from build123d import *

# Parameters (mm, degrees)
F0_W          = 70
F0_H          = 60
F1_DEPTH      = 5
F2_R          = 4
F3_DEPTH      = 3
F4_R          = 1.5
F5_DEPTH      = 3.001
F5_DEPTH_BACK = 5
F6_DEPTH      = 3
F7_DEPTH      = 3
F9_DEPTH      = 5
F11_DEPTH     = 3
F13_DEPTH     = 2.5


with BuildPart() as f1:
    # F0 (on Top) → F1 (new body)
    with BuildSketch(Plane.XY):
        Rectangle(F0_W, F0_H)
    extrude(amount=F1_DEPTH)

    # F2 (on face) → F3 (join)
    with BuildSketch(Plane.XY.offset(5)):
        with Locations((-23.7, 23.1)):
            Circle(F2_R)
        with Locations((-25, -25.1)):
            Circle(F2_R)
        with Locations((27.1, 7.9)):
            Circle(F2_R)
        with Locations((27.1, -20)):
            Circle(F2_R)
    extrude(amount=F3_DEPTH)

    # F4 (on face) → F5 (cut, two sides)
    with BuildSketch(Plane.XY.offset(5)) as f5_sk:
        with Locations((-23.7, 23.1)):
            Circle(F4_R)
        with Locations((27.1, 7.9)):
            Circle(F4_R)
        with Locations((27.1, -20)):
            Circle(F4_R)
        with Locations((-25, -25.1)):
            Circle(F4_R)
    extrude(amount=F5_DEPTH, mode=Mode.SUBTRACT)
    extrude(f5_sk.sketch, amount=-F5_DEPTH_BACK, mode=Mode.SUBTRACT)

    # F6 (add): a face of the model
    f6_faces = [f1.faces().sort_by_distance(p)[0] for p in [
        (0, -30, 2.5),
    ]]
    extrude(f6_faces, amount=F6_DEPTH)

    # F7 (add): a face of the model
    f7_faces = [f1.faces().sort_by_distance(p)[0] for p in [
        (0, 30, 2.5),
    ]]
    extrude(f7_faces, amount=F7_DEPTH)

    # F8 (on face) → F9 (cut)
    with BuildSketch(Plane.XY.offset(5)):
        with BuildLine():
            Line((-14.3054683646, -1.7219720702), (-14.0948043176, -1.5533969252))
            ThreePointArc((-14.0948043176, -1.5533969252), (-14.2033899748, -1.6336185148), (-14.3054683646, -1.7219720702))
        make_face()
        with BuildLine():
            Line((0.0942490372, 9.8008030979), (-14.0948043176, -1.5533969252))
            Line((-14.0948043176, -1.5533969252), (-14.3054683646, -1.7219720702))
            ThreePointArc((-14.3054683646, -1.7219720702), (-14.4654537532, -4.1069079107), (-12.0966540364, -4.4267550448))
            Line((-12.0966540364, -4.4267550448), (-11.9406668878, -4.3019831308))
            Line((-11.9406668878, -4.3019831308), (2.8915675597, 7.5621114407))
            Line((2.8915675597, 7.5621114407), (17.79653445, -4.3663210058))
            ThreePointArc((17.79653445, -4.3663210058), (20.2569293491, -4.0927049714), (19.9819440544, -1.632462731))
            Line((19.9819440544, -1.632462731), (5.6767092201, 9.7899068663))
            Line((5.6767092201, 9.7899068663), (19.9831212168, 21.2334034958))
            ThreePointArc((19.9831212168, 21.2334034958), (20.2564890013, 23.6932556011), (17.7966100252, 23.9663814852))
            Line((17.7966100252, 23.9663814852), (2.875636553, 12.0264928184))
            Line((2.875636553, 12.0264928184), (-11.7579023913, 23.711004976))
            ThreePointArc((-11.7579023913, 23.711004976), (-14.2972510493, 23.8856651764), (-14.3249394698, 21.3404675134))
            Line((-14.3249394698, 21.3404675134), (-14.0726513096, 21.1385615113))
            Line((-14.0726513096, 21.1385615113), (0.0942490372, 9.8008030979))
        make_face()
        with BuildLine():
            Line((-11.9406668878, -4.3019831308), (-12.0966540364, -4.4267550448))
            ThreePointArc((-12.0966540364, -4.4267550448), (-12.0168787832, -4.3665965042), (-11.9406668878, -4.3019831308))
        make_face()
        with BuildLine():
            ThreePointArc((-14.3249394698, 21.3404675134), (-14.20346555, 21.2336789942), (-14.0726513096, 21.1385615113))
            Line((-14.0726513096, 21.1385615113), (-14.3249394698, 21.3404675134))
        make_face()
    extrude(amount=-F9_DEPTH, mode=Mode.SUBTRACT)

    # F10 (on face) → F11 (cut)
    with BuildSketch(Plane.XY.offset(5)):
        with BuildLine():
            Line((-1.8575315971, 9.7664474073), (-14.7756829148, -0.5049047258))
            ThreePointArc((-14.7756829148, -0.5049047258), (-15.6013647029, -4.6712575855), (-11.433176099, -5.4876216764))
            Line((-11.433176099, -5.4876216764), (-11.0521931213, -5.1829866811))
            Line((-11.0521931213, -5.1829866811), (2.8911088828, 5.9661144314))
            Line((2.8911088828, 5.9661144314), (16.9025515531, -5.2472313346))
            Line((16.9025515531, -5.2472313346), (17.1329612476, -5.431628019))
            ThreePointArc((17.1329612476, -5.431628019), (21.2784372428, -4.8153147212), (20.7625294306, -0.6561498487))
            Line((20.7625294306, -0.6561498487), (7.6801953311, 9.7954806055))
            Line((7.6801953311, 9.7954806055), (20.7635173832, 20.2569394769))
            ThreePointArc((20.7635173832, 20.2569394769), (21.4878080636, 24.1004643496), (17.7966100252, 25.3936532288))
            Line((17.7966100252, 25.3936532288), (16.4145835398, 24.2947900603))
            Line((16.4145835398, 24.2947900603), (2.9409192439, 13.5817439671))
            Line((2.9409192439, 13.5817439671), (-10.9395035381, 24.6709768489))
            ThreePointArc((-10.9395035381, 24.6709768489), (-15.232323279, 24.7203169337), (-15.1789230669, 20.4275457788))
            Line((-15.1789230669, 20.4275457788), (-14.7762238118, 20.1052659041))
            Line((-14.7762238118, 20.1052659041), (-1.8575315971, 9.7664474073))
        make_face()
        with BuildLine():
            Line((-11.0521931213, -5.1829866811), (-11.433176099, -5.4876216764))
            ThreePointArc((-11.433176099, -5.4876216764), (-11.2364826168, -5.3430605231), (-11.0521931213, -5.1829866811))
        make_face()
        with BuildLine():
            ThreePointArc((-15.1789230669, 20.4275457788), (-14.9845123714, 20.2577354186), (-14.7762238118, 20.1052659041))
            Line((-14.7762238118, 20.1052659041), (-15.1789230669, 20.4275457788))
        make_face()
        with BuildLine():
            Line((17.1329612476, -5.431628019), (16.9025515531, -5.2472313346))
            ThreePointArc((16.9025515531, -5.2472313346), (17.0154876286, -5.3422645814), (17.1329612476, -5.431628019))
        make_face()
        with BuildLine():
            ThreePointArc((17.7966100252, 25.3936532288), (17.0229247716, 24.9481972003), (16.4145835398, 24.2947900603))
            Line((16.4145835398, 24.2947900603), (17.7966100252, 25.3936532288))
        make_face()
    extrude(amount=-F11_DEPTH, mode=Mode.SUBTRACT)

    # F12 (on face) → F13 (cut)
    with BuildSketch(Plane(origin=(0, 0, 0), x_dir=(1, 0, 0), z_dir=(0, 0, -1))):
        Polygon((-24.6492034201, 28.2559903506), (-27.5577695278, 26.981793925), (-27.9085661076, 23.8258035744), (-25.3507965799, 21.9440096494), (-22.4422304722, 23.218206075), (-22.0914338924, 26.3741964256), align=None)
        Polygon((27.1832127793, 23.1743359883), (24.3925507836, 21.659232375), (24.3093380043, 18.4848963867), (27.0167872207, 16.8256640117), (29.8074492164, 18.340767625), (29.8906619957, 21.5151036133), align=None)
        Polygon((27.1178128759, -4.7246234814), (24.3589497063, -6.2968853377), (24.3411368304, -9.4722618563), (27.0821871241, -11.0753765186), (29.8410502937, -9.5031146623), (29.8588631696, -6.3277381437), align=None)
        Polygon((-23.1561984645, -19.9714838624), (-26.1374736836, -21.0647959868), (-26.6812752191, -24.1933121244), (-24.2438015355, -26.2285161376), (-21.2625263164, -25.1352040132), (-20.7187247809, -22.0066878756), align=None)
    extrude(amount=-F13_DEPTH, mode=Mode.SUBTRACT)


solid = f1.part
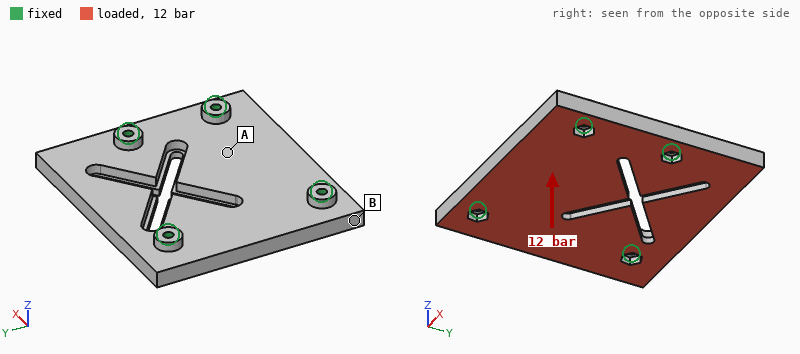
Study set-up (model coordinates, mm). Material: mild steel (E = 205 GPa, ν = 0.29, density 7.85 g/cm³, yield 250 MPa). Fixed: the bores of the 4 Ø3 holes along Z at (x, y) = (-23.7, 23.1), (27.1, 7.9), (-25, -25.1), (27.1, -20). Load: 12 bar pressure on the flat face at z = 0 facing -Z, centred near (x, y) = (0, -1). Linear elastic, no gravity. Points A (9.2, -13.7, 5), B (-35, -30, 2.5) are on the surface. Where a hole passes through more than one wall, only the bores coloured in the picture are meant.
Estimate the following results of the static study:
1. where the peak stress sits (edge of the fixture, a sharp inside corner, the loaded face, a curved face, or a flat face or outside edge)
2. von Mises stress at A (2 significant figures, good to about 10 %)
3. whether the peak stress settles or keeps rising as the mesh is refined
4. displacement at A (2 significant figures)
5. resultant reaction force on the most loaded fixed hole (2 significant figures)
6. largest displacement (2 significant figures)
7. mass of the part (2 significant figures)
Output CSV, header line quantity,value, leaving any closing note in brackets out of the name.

quantity,value
where the peak stress sits,edge of the fixture
von Mises stress at A,31 MPa
whether the peak stress settles or keeps rising as the mesh is refined,keeps rising
displacement at A,19 µm
resultant reaction force on the most loaded fixed hole,1.6 kN
largest displacement,45 µm
mass of the part,170 g
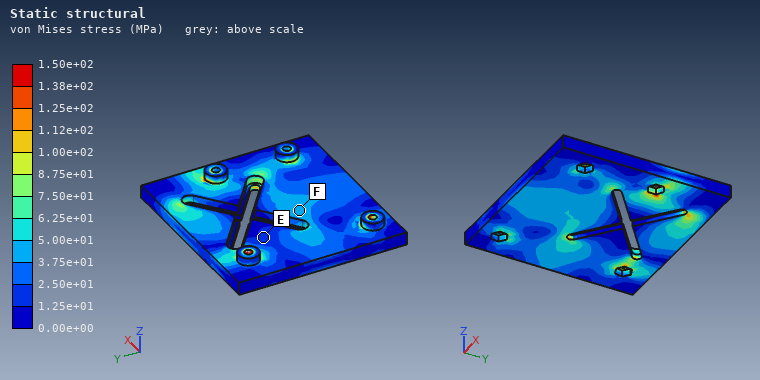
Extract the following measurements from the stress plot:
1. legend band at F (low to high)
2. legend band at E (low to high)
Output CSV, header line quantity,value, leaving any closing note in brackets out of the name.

quantity,value
legend band at F,3.75e+01 to 5.00e+01 MPa
legend band at E,1.25e+01 to 2.50e+01 MPa
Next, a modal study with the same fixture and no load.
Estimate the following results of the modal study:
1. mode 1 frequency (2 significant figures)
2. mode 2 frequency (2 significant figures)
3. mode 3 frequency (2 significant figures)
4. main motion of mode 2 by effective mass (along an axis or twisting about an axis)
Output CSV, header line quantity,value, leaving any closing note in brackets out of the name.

quantity,value
mode 1 frequency,5000 Hz
mode 2 frequency,6000 Hz
mode 3 frequency,7700 Hz
main motion of mode 2 by effective mass,along Z
